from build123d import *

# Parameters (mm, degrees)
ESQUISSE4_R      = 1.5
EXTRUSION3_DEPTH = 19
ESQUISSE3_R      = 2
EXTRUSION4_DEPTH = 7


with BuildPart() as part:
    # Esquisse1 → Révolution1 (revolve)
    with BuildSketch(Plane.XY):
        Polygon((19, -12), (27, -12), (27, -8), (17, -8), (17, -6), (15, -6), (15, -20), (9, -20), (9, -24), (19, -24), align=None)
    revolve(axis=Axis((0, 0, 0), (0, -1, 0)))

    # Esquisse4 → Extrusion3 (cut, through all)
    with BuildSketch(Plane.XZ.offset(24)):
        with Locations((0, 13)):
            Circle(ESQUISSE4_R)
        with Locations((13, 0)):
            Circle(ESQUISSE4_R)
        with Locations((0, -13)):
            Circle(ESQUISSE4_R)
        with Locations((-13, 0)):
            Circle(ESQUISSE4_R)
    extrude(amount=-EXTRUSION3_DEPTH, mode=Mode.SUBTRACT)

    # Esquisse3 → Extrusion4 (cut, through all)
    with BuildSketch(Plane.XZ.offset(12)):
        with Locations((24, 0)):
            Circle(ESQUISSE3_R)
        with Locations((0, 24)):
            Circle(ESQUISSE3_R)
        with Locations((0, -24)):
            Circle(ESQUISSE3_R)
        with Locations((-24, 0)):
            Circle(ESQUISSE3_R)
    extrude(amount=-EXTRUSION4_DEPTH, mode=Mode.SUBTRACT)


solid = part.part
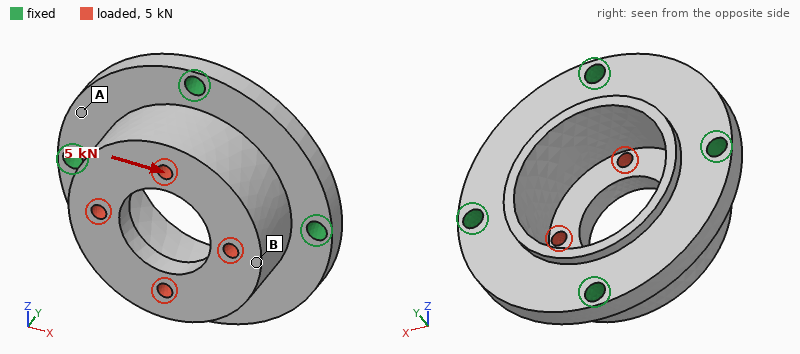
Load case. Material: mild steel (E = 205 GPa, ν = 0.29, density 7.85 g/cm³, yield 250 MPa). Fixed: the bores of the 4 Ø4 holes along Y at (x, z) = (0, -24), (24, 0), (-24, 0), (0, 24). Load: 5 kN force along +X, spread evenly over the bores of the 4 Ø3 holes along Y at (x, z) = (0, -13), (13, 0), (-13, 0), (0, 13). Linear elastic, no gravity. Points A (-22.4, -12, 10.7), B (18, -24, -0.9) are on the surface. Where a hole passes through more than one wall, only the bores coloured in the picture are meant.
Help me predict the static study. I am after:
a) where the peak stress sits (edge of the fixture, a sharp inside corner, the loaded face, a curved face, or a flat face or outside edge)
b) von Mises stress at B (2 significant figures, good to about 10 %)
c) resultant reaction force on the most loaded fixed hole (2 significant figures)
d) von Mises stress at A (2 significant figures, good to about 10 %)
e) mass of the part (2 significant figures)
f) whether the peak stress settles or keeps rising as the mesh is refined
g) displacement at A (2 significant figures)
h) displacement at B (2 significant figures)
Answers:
edge of the fixture
49 MPa
1.8 kN
18 MPa
100 g
keeps rising
3.3 µm
10 µm
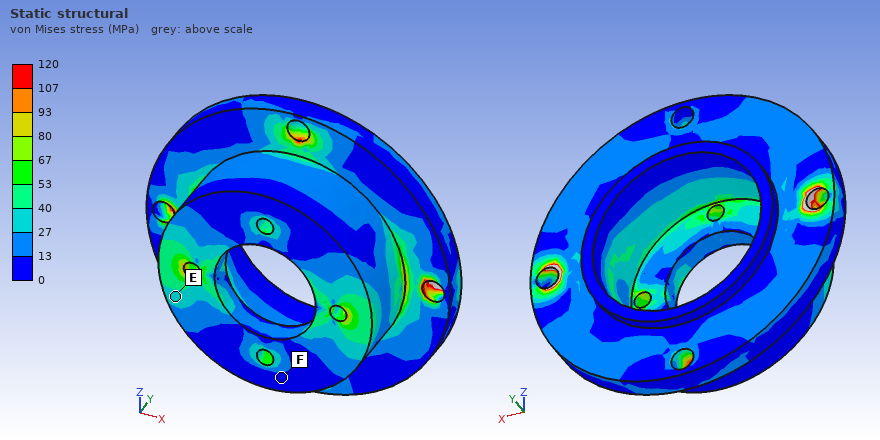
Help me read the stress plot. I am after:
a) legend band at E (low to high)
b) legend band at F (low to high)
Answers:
27 to 40 MPa
0 to 13 MPa
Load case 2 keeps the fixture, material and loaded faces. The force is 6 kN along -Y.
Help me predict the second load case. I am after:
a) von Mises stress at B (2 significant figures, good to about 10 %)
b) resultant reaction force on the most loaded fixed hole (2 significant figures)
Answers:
35 MPa
1.6 kN
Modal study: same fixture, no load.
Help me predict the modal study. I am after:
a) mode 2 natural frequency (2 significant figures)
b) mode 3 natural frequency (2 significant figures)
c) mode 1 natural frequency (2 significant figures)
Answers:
17 kHz
17 kHz
17 kHz
